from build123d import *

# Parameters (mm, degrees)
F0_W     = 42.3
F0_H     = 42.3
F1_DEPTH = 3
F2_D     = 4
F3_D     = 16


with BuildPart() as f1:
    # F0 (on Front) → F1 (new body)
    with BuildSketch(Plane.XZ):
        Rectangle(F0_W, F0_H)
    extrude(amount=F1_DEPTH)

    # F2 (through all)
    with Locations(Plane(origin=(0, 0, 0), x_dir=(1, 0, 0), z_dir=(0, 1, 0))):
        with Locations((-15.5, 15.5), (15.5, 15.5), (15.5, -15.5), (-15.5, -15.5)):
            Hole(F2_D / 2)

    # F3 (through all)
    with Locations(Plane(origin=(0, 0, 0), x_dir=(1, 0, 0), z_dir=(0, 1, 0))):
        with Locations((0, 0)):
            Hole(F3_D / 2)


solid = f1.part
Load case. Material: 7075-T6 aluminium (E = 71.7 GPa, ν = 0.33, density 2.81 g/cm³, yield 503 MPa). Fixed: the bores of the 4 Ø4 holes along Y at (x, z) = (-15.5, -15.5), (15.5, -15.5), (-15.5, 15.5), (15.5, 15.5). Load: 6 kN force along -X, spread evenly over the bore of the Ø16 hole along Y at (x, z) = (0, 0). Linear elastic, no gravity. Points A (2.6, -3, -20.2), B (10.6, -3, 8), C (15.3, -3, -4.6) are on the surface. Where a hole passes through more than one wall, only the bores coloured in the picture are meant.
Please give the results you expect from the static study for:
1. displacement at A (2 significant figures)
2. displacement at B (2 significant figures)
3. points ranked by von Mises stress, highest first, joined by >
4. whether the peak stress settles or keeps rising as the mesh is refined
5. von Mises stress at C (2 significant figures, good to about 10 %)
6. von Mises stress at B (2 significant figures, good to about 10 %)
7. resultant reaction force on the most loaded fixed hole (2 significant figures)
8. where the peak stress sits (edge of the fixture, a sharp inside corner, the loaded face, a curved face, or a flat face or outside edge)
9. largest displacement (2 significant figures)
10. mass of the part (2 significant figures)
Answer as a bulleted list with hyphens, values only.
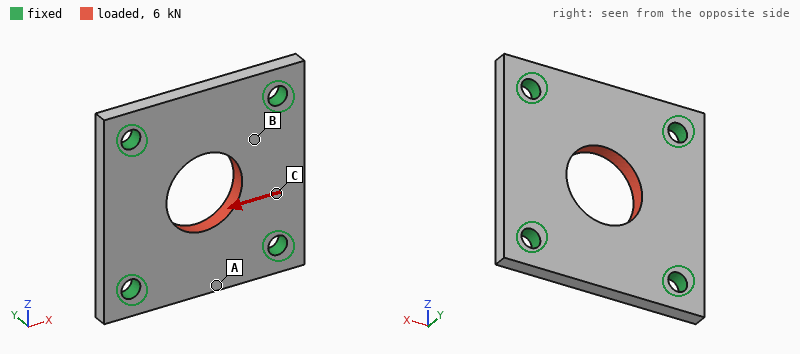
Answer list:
- 2.7 µm
- 8.6 µm
- B > C > A
- keeps rising
- 27 MPa
- 45 MPa
- 1.6 kN
- edge of the fixture
- 15 µm
- 13 g
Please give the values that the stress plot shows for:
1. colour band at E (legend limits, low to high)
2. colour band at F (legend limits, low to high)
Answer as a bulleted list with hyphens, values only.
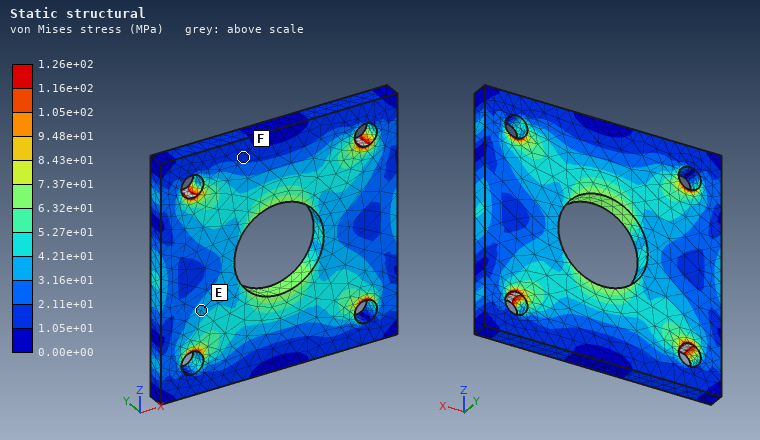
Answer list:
- 3.16e+01 to 4.21e+01 MPa
- 1.05e+01 to 2.11e+01 MPa
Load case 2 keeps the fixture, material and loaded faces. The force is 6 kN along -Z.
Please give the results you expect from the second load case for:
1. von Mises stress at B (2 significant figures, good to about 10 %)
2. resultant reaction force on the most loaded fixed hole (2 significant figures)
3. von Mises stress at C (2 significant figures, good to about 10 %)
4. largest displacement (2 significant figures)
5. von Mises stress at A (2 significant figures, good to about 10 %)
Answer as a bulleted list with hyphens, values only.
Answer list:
- 45 MPa
- 1.6 kN
- 27 MPa
- 15 µm
- 31 MPa
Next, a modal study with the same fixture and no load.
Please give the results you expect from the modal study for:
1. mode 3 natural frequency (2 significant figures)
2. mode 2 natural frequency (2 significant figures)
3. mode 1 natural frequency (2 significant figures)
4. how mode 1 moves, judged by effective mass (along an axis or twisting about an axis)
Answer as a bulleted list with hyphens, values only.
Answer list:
- 18 kHz
- 18 kHz
- 14 kHz
- along Y
